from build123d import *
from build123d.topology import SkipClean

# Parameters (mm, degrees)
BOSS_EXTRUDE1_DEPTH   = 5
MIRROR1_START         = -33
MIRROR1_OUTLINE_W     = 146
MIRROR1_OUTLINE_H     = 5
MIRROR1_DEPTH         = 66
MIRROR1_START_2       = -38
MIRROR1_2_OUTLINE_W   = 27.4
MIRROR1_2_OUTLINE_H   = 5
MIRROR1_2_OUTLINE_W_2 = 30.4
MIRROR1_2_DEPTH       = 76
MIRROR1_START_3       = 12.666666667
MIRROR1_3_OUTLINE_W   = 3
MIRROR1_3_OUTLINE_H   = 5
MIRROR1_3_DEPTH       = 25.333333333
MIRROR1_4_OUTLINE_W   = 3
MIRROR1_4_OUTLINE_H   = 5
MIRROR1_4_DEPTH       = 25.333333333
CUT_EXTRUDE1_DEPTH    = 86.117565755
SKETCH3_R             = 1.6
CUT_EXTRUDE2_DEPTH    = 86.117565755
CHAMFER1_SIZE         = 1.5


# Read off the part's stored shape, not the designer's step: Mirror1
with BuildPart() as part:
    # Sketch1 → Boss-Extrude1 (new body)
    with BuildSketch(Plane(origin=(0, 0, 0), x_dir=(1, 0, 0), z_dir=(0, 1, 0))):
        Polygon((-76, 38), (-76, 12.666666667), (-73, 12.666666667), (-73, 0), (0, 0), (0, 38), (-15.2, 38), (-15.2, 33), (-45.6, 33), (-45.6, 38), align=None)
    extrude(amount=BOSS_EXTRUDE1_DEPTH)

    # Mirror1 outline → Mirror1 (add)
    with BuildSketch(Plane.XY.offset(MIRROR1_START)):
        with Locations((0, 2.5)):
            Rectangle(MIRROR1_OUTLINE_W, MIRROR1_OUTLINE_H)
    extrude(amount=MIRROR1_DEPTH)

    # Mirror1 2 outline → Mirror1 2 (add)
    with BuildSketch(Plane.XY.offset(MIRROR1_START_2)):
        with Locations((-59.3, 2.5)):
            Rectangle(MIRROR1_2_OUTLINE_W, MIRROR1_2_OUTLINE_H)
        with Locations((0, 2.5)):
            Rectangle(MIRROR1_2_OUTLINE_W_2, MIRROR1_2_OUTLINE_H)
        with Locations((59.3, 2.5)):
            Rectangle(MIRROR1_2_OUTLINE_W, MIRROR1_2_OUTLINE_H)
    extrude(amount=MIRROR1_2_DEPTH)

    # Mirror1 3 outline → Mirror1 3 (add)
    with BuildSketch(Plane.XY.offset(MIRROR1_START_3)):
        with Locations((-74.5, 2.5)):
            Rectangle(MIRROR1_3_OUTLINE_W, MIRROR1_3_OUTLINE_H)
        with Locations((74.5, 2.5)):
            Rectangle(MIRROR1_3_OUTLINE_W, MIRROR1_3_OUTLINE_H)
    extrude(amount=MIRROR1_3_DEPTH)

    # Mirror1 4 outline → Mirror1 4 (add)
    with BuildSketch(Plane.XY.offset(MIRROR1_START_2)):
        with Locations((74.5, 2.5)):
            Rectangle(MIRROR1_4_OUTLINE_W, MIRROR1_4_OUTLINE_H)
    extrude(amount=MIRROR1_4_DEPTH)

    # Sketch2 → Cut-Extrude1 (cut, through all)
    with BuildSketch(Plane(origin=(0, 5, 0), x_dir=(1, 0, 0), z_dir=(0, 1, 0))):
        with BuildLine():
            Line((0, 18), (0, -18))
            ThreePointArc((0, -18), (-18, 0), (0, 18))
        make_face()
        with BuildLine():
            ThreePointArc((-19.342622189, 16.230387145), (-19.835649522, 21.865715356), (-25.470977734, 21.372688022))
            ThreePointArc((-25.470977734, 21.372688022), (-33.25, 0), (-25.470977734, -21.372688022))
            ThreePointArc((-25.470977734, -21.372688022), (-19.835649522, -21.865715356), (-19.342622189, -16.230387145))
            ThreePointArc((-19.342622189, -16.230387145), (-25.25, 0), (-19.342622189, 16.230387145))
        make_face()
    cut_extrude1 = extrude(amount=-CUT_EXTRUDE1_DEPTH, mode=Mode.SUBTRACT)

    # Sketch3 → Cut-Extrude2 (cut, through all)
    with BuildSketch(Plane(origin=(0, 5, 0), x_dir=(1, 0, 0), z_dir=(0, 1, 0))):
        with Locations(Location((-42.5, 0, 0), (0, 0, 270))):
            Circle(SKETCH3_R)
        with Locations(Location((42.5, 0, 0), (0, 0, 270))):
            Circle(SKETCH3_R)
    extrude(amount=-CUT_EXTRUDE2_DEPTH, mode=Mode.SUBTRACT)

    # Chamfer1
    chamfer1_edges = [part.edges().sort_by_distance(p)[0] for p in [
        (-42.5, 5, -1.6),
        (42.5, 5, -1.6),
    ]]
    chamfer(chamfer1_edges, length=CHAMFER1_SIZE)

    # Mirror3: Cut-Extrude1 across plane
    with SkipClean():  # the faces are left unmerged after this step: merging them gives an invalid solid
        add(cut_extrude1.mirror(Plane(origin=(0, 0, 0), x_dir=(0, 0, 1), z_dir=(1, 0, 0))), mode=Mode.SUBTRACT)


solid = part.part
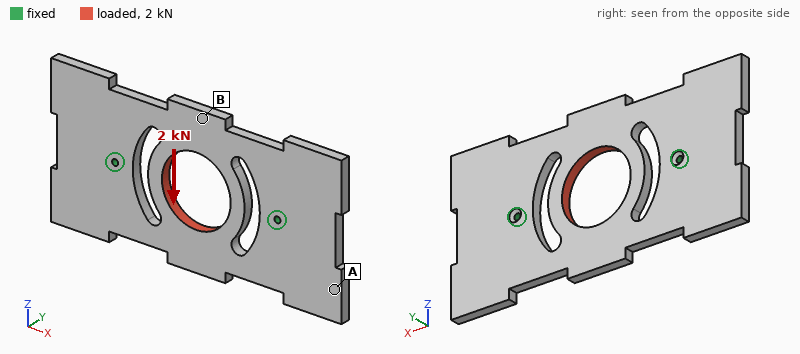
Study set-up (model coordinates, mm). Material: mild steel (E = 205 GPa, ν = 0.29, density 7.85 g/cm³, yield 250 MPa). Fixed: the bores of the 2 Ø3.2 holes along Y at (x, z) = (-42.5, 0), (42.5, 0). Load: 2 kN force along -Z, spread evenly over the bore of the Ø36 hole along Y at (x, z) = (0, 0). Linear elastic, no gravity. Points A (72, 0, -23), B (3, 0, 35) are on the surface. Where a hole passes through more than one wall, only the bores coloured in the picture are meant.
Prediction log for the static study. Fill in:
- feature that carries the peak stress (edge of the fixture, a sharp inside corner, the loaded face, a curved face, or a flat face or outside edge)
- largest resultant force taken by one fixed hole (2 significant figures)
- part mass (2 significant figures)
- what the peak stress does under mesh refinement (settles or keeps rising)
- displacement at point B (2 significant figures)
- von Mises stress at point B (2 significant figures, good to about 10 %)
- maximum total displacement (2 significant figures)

edge of the fixture
1.0 kN
350 g
keeps rising
7.1 µm
13 MPa
7.6 µm
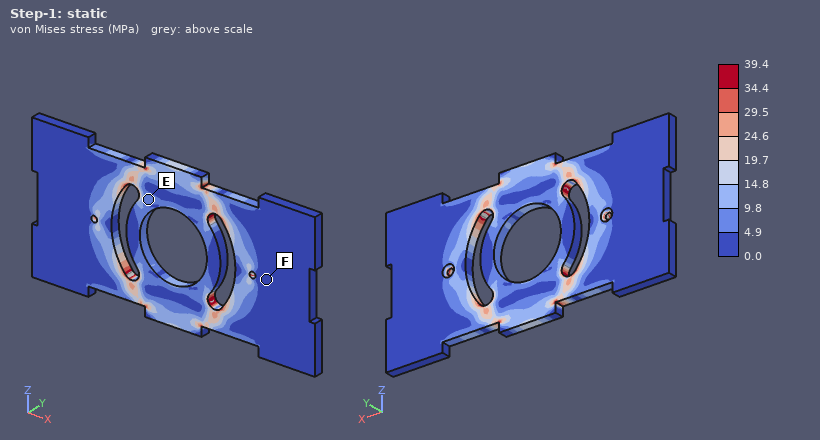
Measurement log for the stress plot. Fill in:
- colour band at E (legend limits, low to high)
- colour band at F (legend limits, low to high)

4.9 to 9.8 MPa
0.0 to 4.9 MPa
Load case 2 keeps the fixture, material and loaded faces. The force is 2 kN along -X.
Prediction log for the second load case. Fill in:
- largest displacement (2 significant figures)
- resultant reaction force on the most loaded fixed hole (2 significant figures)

5.7 µm
1.0 kN
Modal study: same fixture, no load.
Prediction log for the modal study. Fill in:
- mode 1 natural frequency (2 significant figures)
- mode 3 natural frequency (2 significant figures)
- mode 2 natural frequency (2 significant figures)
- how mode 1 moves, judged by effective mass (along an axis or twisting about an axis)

1200 Hz
1700 Hz
1600 Hz
twisting about X
